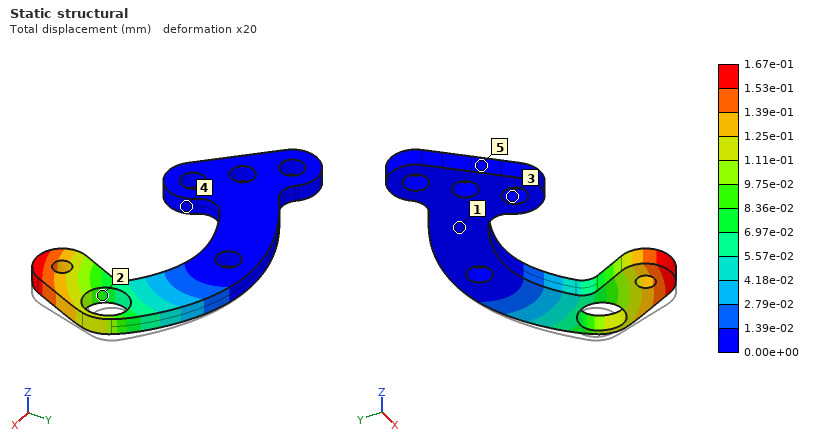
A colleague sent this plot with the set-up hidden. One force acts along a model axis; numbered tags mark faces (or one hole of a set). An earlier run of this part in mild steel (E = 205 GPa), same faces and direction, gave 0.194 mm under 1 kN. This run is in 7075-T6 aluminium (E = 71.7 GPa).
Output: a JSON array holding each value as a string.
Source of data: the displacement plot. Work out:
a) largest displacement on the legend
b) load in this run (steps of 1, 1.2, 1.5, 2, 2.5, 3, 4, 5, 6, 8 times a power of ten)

["1.67e-01 mm", "300 N"]
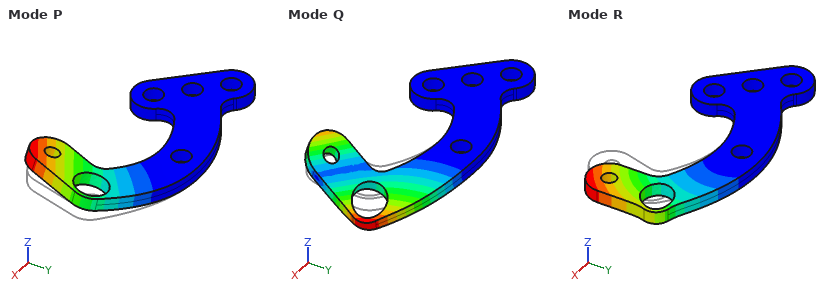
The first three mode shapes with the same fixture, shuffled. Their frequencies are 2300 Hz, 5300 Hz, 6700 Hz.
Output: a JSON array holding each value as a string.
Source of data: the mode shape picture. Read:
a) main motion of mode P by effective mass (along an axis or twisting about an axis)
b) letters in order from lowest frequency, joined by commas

["along Z", "P, R, Q"]
